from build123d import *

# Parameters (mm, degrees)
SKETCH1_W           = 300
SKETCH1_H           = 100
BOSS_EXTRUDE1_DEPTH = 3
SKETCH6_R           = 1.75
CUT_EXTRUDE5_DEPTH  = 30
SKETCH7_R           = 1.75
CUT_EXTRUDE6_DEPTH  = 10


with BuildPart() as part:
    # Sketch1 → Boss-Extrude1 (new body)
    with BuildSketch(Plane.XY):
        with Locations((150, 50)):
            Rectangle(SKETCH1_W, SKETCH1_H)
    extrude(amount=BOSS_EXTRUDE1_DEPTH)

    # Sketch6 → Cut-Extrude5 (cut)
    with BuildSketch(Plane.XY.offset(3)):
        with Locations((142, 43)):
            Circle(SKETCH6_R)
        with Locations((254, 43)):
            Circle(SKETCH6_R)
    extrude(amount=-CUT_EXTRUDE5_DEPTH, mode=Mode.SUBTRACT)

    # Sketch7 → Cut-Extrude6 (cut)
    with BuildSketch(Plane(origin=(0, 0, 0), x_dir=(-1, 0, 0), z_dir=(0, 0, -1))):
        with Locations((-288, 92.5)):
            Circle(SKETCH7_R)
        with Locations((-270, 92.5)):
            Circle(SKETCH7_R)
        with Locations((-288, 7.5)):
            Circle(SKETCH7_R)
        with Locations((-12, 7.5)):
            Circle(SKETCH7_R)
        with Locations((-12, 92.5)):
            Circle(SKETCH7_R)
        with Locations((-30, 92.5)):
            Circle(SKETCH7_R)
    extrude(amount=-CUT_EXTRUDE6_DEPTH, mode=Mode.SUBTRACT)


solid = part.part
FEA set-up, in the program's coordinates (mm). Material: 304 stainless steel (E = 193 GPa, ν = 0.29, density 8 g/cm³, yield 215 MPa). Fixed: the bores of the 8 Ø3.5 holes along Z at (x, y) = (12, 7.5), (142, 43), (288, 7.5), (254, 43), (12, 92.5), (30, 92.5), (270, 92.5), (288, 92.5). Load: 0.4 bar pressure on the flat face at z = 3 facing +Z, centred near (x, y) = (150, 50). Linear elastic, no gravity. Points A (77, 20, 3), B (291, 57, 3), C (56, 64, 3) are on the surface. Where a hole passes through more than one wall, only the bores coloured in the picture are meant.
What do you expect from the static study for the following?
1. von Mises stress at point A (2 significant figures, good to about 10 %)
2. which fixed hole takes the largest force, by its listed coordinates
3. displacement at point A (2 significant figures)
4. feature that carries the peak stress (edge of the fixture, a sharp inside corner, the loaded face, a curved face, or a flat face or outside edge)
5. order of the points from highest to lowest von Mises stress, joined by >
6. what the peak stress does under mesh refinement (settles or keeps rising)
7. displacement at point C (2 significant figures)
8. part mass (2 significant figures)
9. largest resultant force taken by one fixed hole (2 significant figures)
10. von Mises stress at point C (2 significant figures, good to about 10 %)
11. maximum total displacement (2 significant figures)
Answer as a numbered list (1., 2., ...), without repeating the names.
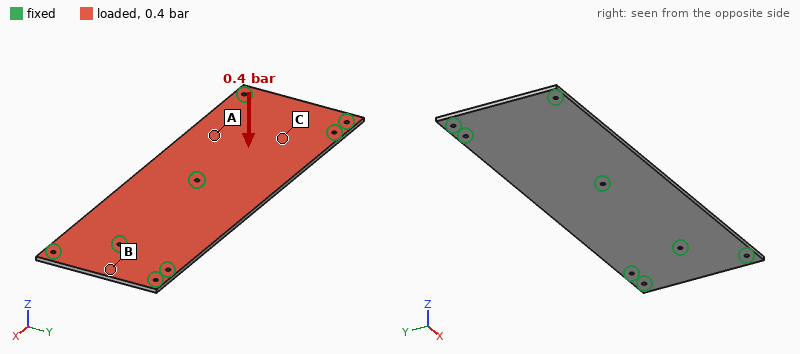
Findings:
1. 17 MPa
2. (142, 43)
3. 0.080 mm
4. edge of the fixture
5. A > C > B
6. keeps rising
7. 0.054 mm
8. 720 g
9. 480 N
10. 11 MPa
11. 0.13 mm
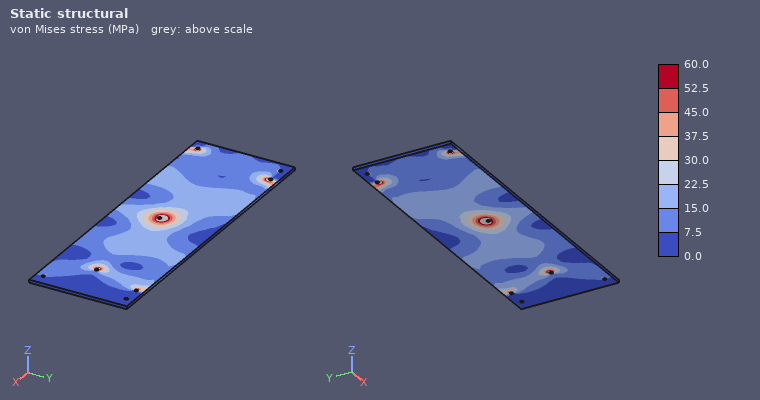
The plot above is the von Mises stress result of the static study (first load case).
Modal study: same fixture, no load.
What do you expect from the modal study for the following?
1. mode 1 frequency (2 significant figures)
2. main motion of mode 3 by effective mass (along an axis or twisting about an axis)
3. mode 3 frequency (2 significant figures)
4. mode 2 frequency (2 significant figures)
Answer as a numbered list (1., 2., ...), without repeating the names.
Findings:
1. 640 Hz
2. along Z
3. 860 Hz
4. 770 Hz
